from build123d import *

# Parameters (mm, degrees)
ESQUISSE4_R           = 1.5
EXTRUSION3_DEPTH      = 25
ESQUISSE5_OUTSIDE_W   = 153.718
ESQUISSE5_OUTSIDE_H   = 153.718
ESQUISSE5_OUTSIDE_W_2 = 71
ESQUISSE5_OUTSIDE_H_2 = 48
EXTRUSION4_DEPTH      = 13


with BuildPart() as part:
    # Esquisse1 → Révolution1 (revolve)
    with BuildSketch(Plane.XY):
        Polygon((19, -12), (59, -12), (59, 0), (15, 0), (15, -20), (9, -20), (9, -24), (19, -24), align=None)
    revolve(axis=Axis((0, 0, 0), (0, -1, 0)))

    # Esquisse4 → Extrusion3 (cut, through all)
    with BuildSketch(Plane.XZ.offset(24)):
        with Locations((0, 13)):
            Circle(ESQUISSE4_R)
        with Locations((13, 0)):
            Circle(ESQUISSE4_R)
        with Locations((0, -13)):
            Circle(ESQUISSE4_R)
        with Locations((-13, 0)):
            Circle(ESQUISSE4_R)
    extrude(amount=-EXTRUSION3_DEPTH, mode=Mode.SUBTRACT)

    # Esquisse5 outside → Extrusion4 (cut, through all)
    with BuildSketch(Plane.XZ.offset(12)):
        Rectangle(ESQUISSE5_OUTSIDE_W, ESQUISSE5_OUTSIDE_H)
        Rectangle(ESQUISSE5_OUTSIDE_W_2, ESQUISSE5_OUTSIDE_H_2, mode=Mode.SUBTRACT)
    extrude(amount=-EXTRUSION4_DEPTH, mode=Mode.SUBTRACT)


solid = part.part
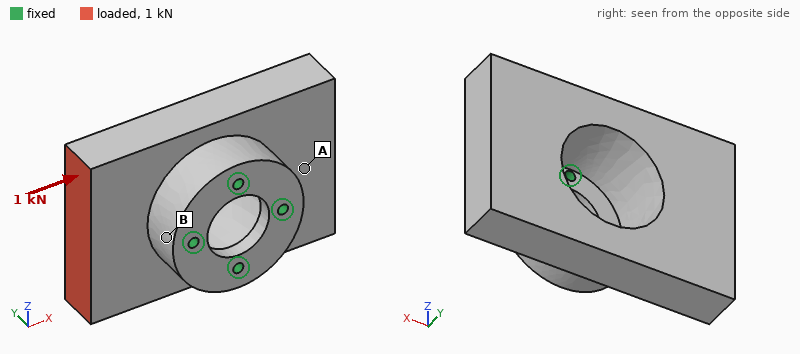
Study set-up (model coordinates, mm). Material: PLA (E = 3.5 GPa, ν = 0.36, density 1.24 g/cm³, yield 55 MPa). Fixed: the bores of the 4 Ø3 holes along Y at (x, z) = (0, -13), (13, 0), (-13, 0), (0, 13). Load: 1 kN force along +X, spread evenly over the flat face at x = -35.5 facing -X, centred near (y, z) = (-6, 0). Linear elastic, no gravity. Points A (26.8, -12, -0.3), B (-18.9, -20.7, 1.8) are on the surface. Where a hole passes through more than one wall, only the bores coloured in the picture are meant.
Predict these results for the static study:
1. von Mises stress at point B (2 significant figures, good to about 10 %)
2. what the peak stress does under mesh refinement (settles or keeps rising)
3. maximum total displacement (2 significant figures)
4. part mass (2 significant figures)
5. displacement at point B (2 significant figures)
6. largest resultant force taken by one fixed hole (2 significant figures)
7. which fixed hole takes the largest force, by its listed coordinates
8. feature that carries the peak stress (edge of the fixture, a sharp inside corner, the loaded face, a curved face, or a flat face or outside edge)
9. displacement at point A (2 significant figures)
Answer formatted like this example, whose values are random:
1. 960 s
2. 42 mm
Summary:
1. 5.7 MPa
2. keeps rising
3. 0.28 mm
4. 49 g
5. 0.082 mm
6. 520 N
7. (-13, 0)
8. edge of the fixture
9. 0.14 mm
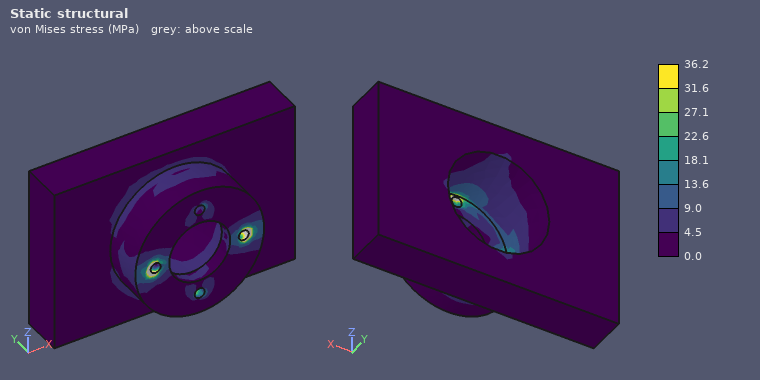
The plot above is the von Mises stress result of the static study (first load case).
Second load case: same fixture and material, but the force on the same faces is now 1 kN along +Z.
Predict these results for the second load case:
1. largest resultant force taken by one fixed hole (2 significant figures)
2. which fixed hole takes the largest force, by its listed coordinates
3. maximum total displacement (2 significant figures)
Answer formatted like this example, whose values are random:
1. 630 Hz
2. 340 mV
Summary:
1. 1.1 kN
2. (-13, 0)
3. 0.40 mm
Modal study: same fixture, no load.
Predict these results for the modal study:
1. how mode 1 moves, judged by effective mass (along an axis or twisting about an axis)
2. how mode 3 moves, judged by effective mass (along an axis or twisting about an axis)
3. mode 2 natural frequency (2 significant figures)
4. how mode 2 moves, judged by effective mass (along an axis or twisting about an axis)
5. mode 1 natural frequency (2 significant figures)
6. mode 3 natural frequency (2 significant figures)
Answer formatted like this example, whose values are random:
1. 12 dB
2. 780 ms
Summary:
1. along X
2. twisting about Y
3. 1800 Hz
4. along Z
5. 1500 Hz
6. 2600 Hz
